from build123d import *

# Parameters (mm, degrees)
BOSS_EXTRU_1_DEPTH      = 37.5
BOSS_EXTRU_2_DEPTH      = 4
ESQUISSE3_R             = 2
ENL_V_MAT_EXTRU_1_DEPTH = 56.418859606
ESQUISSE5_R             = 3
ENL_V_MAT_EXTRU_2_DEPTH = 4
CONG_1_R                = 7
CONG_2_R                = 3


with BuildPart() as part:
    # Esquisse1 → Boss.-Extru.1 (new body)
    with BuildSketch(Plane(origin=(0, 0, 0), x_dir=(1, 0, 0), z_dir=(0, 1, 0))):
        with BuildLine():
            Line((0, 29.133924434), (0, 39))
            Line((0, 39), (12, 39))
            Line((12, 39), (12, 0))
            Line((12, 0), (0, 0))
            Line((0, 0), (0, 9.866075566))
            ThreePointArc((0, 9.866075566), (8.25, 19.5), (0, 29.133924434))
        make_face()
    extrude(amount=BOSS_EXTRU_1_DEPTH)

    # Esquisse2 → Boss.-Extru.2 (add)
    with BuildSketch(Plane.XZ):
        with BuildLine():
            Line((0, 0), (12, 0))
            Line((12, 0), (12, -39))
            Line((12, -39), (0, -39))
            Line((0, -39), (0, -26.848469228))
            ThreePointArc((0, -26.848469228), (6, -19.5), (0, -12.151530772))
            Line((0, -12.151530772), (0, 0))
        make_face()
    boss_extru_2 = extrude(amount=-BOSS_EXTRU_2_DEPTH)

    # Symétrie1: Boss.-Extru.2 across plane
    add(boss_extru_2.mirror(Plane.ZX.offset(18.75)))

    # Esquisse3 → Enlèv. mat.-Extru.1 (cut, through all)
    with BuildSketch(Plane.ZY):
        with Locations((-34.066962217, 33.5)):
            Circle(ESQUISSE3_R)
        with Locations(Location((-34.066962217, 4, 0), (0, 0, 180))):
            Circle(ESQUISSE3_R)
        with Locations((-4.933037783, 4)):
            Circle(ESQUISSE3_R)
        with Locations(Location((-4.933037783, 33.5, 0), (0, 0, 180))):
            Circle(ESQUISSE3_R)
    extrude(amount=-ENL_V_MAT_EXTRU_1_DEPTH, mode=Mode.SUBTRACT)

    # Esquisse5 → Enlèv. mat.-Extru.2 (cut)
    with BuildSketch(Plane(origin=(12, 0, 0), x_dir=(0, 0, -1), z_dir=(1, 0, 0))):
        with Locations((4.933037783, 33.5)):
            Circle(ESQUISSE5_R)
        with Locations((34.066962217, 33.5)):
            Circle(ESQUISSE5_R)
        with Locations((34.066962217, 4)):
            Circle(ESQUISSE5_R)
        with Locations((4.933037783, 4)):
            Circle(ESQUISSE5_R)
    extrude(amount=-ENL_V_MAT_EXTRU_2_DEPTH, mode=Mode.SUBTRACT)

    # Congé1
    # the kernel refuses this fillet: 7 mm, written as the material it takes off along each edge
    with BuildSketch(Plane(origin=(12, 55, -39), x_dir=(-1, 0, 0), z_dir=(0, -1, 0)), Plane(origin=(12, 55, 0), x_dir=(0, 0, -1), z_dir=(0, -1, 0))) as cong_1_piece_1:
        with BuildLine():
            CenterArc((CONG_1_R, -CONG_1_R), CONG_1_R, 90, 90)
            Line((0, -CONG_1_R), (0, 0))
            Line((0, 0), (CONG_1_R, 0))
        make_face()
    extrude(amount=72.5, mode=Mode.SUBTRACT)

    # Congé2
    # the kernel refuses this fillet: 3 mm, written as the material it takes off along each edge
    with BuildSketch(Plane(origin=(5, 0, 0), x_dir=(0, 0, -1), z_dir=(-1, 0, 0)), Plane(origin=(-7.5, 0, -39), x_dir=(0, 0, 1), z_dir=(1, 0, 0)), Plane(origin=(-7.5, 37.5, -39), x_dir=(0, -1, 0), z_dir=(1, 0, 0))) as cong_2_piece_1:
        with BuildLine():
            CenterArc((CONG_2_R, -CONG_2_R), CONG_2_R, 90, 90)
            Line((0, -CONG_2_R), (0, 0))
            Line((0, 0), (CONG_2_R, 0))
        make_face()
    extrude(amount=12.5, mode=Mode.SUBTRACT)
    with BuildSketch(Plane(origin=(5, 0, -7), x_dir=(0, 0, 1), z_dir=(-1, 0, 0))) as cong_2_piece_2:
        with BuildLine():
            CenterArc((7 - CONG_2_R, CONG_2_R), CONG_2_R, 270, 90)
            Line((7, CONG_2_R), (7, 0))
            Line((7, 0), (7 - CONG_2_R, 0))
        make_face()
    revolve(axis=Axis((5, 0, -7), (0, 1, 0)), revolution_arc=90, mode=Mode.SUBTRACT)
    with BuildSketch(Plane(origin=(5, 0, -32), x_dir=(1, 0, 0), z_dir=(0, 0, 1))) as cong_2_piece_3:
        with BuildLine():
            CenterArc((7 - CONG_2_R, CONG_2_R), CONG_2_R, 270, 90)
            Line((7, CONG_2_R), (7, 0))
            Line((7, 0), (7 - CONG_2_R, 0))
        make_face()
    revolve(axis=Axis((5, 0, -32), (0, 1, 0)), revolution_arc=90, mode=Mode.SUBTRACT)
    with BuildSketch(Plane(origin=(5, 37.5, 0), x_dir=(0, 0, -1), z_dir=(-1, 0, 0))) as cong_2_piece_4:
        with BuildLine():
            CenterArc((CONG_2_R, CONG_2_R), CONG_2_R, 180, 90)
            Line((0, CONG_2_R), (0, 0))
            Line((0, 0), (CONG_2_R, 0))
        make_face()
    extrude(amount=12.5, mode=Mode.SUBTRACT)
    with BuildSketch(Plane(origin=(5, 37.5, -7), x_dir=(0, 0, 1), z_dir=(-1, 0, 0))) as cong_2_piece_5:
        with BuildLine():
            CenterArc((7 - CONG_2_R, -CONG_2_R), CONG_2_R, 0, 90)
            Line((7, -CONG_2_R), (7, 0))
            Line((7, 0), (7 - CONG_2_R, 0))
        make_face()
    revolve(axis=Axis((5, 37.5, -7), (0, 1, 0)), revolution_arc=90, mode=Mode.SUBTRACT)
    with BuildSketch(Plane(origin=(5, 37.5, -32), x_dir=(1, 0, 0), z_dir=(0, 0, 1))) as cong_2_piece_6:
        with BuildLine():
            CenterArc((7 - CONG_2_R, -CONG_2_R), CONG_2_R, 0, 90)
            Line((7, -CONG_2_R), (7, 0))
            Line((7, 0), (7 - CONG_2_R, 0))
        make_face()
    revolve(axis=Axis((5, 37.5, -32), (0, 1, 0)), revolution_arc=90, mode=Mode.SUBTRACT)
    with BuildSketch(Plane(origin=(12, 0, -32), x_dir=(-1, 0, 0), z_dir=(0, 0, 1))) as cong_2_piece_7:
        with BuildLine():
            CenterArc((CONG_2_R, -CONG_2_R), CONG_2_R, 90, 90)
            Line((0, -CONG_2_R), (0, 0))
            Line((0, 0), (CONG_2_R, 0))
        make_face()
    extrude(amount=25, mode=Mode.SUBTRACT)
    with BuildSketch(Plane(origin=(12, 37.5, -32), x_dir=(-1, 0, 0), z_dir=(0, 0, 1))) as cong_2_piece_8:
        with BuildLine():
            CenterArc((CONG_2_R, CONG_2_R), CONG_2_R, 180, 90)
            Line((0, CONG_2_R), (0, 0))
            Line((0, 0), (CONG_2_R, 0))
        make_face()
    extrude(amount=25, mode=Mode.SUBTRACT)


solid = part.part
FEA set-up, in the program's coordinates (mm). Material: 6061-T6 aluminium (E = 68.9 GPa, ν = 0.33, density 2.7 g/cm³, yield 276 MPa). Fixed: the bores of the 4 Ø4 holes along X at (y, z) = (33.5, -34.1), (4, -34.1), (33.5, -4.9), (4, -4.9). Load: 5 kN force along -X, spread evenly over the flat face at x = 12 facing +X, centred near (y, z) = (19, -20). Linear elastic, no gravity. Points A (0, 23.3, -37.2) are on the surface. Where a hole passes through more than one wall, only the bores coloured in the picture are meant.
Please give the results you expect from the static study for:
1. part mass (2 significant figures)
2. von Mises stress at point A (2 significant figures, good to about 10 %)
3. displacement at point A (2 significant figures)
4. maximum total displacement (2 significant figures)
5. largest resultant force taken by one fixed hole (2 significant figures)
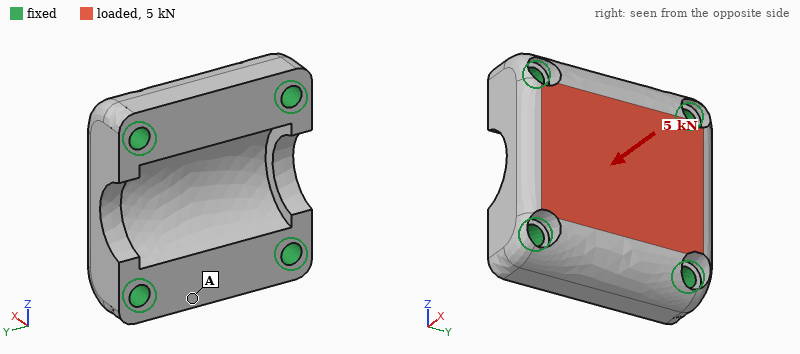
32 g
12 MPa
4.3 µm
13 µm
1.7 kN
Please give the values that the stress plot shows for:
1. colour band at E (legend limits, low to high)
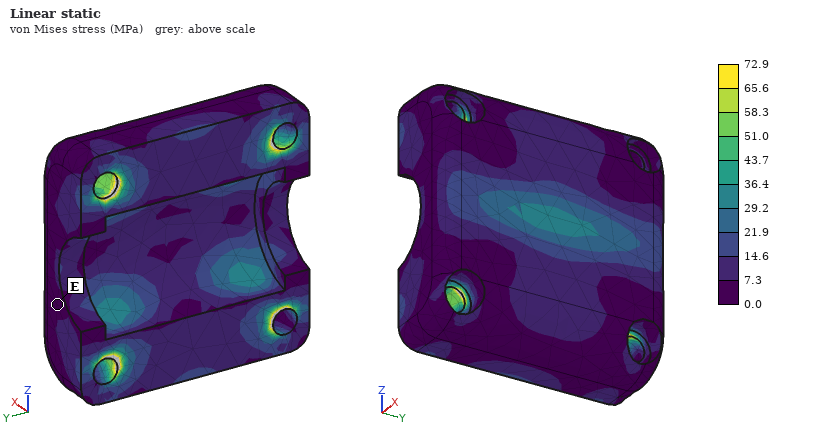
0.0 to 7.3 MPa
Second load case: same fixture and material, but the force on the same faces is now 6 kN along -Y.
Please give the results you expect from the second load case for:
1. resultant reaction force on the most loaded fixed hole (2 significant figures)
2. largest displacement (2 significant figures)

1.8 kN
7.3 µm
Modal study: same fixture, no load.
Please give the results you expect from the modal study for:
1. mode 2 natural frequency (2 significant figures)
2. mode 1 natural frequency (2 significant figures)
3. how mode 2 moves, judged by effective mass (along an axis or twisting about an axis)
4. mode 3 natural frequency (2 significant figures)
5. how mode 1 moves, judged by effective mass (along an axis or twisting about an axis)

35 kHz
31 kHz
along Z
40 kHz
along X
